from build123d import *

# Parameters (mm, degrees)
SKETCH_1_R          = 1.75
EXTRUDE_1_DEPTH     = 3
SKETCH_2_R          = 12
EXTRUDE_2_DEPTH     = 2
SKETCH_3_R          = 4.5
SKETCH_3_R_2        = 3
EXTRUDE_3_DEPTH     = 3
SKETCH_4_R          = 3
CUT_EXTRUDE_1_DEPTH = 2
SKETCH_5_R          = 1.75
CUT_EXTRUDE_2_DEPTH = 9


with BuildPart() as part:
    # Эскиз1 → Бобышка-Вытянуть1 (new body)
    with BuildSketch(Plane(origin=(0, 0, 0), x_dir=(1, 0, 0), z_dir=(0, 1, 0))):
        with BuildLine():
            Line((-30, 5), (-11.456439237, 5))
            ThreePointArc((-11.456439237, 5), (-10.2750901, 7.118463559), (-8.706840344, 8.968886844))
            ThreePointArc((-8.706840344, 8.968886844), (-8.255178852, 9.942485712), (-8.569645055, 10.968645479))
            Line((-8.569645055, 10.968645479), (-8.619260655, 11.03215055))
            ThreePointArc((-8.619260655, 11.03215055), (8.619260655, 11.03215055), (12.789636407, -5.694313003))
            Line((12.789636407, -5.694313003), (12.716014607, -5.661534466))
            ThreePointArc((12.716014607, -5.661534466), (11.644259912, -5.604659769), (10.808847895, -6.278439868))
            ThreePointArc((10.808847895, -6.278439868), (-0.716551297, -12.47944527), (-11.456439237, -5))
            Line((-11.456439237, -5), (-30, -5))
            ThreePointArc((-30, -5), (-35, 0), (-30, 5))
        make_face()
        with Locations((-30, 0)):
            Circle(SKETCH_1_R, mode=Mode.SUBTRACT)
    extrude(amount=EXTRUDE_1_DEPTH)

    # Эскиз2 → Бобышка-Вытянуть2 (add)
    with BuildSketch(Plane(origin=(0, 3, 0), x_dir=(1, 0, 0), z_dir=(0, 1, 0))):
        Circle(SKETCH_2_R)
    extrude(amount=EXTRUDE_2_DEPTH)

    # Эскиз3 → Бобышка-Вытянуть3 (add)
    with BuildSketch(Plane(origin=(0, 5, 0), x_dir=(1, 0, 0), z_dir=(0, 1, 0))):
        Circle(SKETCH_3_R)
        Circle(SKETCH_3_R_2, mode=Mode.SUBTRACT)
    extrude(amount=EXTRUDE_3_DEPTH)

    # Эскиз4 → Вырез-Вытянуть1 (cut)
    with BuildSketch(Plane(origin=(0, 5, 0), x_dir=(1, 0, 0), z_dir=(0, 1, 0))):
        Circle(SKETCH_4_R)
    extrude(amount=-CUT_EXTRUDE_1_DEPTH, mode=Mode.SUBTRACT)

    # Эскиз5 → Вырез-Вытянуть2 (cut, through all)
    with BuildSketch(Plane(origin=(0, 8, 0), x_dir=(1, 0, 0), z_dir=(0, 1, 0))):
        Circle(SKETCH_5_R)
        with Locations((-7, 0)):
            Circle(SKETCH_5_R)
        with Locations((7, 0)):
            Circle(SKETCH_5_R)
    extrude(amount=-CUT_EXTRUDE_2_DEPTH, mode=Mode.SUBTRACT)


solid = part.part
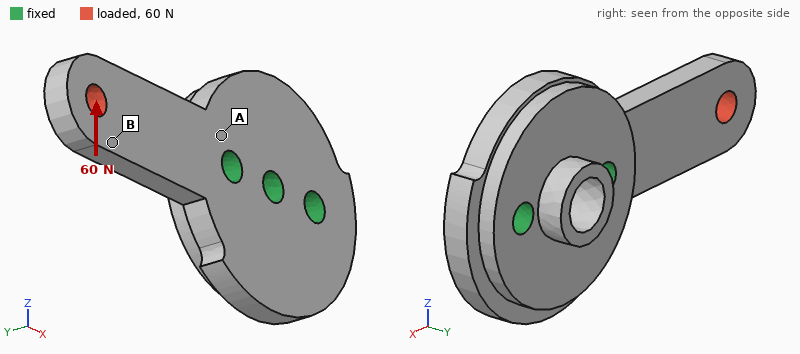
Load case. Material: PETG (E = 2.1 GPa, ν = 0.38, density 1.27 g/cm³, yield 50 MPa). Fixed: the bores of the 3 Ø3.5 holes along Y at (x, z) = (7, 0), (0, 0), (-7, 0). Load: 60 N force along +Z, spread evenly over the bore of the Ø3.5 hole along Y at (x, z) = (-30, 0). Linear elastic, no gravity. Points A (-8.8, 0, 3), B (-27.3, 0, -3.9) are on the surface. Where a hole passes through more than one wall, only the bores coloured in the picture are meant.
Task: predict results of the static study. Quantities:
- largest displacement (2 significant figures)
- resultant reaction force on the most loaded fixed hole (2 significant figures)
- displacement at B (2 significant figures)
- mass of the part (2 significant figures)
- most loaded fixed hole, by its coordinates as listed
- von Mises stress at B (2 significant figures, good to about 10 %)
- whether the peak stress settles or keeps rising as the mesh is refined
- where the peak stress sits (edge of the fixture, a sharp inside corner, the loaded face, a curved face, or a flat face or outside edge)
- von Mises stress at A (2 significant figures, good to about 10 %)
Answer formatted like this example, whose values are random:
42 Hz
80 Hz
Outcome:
0.59 mm
120 N
0.37 mm
3.9 g
(-7, 0)
3.5 MPa
keeps rising
a sharp inside corner
9.3 MPa
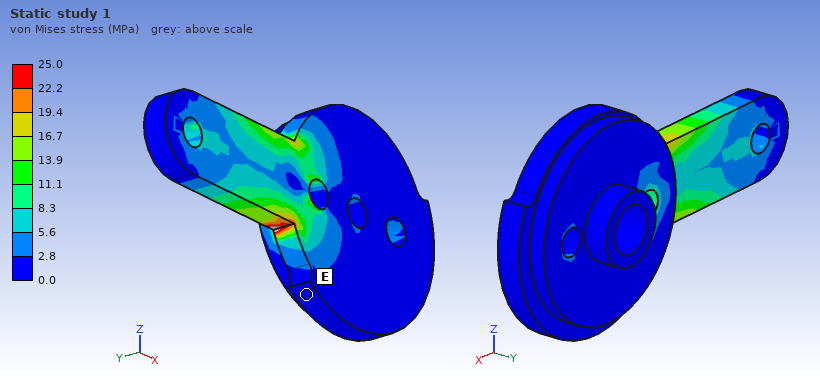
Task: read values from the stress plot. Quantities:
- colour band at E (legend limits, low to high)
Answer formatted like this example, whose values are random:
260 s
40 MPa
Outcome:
0.0 to 2.8 MPa
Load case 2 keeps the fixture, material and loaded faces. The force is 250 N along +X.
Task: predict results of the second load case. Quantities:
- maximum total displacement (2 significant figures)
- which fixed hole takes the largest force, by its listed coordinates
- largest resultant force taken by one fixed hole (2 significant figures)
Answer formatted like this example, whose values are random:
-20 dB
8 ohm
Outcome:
0.14 mm
(-7, 0)
210 N
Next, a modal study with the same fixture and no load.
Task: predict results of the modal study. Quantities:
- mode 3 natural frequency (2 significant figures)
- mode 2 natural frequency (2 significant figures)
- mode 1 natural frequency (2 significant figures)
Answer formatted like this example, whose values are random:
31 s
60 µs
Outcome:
4700 Hz
3000 Hz
1200 Hz
